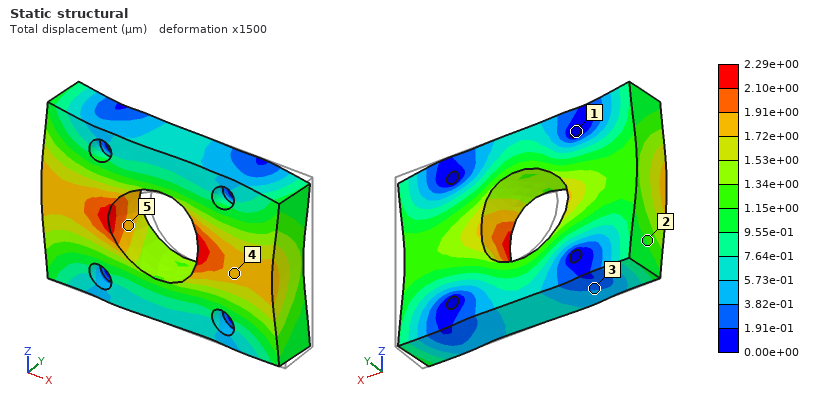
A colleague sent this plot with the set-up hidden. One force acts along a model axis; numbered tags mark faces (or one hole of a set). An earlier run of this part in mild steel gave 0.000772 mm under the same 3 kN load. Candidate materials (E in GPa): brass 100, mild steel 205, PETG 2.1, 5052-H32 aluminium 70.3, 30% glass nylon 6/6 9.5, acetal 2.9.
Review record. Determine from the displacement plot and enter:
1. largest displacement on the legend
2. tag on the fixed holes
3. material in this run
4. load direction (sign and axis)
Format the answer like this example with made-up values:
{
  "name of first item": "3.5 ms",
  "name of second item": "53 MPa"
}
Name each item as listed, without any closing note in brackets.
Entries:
{
  "largest displacement on the legend": "2.29e+00 µm",
  "tag on the fixed holes": "1",
  "material in this run": "5052-H32 aluminium",
  "load direction": "-X"
}
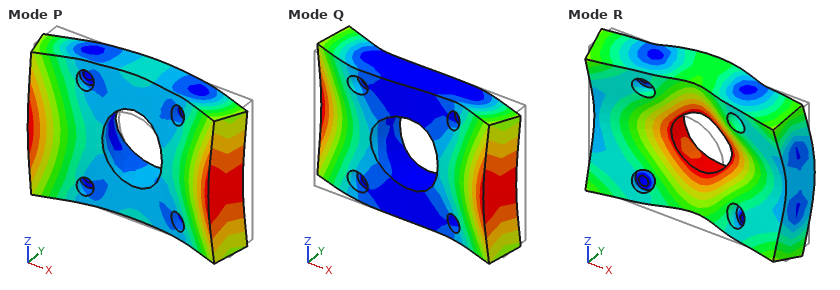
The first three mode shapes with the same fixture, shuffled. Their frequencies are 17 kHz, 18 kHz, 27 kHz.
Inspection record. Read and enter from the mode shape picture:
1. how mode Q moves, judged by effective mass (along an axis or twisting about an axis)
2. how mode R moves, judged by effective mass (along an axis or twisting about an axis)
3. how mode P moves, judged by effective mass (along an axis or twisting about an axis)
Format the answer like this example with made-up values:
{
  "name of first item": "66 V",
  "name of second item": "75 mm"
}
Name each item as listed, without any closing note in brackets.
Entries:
{
  "how mode Q moves, judged by effective mass": "twisting about Z",
  "how mode R moves, judged by effective mass": "along Y",
  "how mode P moves, judged by effective mass": "along Y"
}
